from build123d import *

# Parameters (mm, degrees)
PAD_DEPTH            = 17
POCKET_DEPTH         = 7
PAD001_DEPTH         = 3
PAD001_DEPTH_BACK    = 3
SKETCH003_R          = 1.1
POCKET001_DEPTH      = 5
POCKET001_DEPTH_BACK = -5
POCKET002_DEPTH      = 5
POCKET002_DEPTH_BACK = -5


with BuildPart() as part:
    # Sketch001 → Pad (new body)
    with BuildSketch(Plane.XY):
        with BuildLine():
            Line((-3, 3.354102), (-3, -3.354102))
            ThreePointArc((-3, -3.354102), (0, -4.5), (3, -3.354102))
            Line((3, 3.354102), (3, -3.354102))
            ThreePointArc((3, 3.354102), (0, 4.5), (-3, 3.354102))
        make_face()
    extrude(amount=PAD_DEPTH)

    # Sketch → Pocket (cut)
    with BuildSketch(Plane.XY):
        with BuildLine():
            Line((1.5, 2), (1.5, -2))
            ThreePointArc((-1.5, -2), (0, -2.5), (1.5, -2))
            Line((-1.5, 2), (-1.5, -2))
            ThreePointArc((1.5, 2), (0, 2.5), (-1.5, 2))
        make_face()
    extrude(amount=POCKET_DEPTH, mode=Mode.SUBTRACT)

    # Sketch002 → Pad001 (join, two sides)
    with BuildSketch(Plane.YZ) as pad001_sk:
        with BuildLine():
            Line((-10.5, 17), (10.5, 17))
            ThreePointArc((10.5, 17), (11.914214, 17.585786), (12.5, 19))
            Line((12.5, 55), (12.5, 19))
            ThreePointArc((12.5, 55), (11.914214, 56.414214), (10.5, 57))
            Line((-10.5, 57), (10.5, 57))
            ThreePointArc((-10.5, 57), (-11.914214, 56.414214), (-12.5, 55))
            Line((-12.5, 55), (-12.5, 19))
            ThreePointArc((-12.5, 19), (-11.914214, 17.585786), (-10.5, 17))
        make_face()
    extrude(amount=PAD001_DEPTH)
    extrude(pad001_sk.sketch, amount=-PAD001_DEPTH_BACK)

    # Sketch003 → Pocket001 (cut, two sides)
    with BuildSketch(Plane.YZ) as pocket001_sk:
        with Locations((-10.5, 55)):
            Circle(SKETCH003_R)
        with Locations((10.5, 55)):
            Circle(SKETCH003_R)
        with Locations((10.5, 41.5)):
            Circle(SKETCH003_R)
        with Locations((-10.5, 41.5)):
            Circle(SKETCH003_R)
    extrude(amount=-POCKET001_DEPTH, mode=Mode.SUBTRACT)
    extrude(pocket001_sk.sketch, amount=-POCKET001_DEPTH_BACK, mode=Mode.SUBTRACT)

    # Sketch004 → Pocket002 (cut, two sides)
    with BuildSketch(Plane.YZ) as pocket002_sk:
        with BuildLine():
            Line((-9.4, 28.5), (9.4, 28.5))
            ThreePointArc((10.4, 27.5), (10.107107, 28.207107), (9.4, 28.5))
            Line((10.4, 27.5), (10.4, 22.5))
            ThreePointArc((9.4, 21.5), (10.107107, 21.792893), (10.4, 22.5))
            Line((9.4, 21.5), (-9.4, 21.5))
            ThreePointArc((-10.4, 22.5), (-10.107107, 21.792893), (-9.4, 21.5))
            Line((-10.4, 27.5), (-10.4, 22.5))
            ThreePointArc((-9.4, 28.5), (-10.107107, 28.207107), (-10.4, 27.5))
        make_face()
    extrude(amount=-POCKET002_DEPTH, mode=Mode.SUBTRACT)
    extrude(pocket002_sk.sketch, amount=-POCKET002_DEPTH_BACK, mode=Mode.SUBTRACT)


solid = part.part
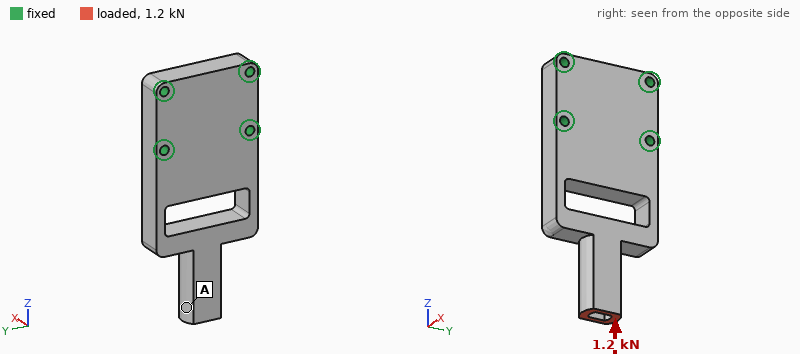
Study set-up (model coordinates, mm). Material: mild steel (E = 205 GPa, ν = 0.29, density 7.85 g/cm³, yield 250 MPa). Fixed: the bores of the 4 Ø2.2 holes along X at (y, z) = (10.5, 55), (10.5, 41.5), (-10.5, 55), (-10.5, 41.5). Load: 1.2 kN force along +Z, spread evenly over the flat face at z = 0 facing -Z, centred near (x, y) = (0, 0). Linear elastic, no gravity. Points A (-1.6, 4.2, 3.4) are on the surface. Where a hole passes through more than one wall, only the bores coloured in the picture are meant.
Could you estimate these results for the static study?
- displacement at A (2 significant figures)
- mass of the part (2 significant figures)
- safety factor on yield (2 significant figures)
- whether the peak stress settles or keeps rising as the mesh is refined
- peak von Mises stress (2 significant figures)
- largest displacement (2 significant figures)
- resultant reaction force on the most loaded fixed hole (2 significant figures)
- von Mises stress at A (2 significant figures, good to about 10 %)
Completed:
19 µm
45 g
0.96
settles
260 MPa
20 µm
560 N
33 MPa
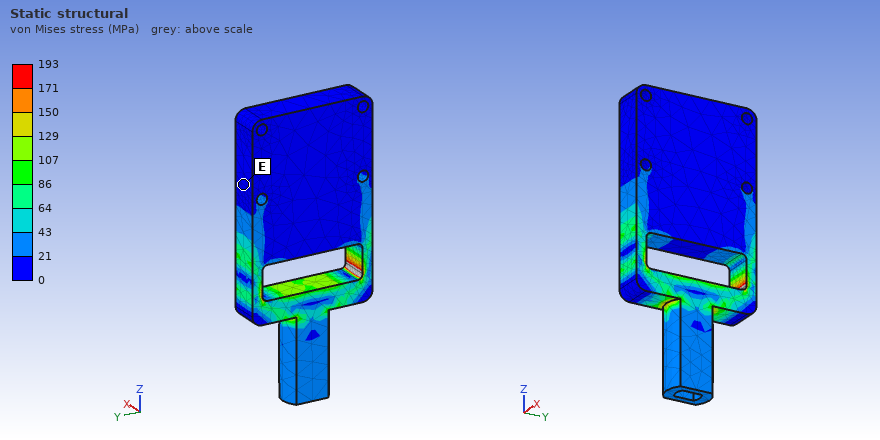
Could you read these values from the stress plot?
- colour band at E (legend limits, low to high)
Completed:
0 to 21 MPa
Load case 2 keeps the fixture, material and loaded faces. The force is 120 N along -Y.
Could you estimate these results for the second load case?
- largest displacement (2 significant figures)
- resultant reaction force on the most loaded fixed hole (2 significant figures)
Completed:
15 µm
230 N
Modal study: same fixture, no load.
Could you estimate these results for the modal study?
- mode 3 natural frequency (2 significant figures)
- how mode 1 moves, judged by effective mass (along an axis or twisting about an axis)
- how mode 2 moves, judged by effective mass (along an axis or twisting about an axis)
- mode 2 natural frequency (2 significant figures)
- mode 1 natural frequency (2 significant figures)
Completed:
12 kHz
along X
along Y
7000 Hz
3000 Hz
